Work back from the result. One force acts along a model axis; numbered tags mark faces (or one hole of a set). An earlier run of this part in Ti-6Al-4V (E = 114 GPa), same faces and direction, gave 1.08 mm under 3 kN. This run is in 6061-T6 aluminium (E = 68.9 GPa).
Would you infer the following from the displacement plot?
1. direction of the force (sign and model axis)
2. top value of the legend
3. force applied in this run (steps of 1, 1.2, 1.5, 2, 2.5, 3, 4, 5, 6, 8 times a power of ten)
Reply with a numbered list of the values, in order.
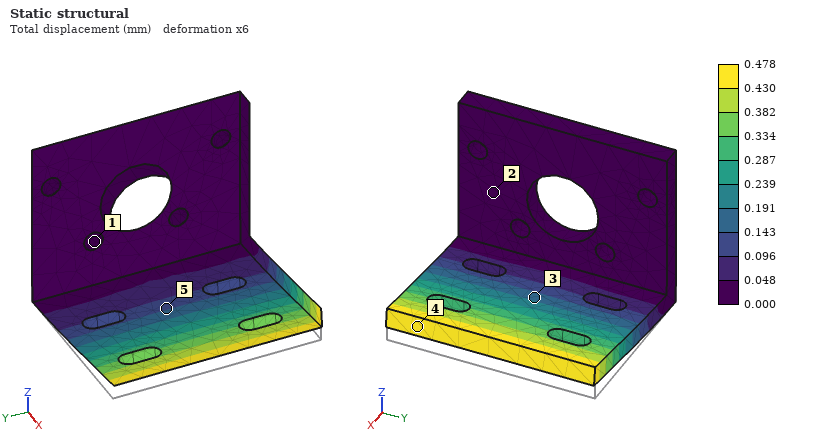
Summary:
1. +Z
2. 0.478 mm
3. 800 N
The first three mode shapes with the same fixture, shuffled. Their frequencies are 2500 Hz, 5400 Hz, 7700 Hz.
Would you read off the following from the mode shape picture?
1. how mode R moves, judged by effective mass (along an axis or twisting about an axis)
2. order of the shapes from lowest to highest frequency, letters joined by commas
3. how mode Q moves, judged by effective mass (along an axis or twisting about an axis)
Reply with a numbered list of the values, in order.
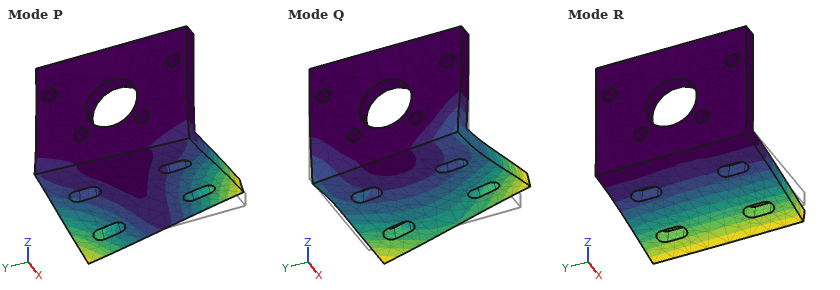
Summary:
1. along Z
2. R, P, Q
3. along Y
